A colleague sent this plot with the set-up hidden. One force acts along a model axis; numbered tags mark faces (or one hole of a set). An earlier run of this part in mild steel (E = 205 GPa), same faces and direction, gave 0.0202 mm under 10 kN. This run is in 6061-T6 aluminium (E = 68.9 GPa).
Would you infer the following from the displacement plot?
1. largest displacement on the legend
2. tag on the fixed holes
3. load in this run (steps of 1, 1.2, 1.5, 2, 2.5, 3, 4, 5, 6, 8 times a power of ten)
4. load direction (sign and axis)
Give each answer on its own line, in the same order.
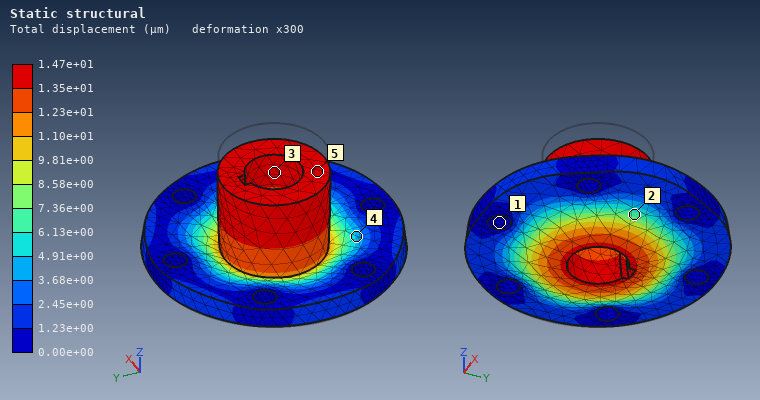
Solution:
1.47e+01 µm
1
2.5 kN
-Z
